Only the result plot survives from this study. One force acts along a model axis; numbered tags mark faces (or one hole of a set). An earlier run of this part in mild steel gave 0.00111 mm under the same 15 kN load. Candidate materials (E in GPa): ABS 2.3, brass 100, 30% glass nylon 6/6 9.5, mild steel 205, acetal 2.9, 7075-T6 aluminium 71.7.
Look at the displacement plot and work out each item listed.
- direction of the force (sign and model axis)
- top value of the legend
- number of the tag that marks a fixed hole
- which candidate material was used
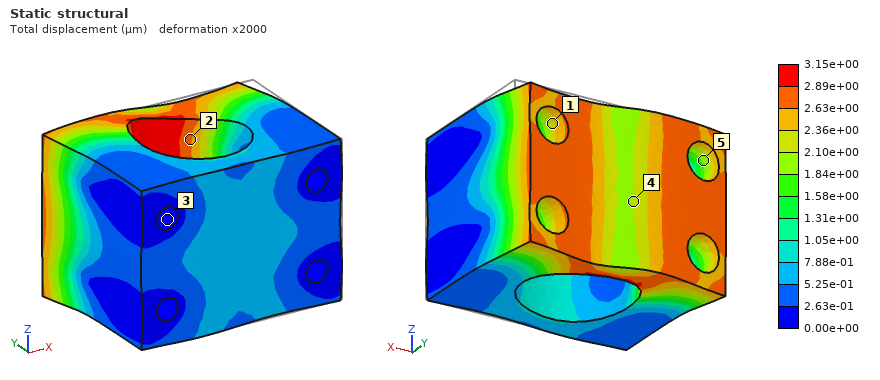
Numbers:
-X
3.15e+00 µm
3
7075-T6 aluminium
